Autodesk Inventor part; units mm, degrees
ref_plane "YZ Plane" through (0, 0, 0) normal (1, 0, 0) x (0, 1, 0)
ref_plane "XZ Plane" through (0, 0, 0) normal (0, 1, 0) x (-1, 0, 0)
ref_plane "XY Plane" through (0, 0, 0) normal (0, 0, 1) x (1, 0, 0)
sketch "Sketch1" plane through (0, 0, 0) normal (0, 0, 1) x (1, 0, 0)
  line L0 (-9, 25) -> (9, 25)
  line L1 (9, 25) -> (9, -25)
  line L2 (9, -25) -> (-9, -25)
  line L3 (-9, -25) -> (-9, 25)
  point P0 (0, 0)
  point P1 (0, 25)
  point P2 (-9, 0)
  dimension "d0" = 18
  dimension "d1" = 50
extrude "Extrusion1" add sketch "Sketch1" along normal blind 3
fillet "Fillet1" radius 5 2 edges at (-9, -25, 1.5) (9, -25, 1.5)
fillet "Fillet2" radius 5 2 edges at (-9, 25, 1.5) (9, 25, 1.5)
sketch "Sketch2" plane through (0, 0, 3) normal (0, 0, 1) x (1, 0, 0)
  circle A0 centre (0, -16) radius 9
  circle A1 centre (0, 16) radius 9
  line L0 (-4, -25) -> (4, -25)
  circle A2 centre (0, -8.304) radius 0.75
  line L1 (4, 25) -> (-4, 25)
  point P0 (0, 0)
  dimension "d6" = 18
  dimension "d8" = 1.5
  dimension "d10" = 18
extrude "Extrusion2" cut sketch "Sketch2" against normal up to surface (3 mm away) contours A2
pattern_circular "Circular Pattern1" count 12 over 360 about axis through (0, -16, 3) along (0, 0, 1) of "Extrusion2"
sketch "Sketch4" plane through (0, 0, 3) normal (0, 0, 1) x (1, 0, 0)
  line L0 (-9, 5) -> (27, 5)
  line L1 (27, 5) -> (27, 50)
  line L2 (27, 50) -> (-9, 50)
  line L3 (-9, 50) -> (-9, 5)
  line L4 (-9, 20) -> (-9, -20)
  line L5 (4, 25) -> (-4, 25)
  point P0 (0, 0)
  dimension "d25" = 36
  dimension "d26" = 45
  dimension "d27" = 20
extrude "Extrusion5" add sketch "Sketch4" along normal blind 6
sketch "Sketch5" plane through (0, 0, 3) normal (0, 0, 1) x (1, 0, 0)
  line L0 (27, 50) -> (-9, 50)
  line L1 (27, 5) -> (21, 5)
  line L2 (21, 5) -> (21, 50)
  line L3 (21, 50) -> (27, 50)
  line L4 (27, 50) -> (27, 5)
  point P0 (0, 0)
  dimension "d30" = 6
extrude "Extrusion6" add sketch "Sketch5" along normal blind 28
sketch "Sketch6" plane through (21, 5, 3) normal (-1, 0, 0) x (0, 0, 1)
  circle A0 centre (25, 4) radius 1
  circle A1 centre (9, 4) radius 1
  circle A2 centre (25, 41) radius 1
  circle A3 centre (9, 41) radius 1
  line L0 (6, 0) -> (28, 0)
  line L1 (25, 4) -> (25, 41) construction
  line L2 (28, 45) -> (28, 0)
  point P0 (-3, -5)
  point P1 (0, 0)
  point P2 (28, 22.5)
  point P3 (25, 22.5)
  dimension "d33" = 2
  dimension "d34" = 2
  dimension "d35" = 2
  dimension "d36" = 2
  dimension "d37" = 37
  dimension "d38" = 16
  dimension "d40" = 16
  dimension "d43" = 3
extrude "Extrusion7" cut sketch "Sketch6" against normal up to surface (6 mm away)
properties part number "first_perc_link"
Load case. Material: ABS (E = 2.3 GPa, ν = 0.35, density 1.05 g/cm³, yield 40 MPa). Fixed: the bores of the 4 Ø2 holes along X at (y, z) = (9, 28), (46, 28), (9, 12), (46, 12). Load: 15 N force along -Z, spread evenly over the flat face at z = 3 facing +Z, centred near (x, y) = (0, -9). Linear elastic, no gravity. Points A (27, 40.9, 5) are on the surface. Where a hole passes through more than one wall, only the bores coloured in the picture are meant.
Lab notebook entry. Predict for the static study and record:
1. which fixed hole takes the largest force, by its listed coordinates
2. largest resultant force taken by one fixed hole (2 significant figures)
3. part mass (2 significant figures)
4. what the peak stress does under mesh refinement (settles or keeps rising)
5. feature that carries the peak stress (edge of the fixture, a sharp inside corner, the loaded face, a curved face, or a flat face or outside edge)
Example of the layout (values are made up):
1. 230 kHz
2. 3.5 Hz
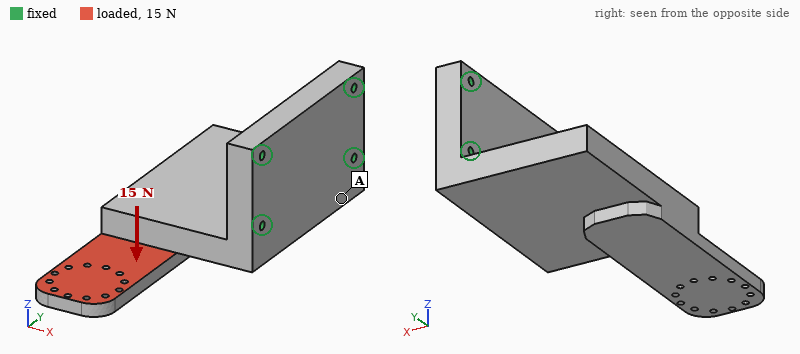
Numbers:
1. (9, 12)
2. 21 N
3. 19 g
4. keeps rising
5. edge of the fixture
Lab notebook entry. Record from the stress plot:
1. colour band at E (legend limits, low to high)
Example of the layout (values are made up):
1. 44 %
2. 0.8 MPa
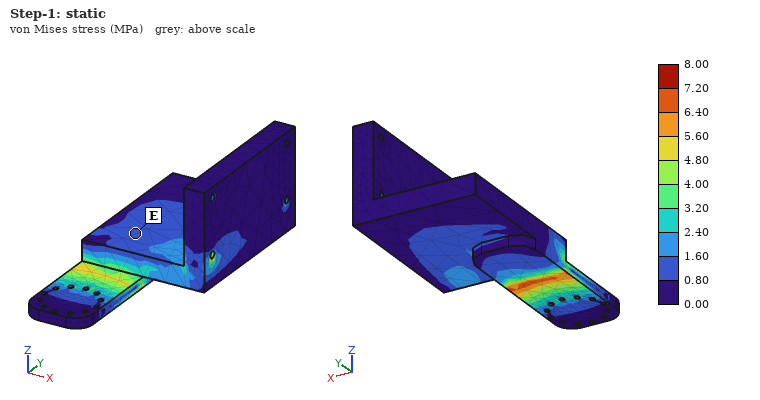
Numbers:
1. 0.80 to 1.60 MPa
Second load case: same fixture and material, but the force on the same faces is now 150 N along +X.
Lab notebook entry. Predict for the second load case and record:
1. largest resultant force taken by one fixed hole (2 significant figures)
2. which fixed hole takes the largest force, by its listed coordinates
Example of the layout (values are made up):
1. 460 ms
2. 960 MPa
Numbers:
1. 250 N
2. (9, 12)
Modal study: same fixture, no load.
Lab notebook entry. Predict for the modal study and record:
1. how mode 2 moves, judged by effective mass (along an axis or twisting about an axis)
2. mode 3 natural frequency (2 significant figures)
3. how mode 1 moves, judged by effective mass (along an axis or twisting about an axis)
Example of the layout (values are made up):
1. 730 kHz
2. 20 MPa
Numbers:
1. along Z
2. 1900 Hz
3. along Z
